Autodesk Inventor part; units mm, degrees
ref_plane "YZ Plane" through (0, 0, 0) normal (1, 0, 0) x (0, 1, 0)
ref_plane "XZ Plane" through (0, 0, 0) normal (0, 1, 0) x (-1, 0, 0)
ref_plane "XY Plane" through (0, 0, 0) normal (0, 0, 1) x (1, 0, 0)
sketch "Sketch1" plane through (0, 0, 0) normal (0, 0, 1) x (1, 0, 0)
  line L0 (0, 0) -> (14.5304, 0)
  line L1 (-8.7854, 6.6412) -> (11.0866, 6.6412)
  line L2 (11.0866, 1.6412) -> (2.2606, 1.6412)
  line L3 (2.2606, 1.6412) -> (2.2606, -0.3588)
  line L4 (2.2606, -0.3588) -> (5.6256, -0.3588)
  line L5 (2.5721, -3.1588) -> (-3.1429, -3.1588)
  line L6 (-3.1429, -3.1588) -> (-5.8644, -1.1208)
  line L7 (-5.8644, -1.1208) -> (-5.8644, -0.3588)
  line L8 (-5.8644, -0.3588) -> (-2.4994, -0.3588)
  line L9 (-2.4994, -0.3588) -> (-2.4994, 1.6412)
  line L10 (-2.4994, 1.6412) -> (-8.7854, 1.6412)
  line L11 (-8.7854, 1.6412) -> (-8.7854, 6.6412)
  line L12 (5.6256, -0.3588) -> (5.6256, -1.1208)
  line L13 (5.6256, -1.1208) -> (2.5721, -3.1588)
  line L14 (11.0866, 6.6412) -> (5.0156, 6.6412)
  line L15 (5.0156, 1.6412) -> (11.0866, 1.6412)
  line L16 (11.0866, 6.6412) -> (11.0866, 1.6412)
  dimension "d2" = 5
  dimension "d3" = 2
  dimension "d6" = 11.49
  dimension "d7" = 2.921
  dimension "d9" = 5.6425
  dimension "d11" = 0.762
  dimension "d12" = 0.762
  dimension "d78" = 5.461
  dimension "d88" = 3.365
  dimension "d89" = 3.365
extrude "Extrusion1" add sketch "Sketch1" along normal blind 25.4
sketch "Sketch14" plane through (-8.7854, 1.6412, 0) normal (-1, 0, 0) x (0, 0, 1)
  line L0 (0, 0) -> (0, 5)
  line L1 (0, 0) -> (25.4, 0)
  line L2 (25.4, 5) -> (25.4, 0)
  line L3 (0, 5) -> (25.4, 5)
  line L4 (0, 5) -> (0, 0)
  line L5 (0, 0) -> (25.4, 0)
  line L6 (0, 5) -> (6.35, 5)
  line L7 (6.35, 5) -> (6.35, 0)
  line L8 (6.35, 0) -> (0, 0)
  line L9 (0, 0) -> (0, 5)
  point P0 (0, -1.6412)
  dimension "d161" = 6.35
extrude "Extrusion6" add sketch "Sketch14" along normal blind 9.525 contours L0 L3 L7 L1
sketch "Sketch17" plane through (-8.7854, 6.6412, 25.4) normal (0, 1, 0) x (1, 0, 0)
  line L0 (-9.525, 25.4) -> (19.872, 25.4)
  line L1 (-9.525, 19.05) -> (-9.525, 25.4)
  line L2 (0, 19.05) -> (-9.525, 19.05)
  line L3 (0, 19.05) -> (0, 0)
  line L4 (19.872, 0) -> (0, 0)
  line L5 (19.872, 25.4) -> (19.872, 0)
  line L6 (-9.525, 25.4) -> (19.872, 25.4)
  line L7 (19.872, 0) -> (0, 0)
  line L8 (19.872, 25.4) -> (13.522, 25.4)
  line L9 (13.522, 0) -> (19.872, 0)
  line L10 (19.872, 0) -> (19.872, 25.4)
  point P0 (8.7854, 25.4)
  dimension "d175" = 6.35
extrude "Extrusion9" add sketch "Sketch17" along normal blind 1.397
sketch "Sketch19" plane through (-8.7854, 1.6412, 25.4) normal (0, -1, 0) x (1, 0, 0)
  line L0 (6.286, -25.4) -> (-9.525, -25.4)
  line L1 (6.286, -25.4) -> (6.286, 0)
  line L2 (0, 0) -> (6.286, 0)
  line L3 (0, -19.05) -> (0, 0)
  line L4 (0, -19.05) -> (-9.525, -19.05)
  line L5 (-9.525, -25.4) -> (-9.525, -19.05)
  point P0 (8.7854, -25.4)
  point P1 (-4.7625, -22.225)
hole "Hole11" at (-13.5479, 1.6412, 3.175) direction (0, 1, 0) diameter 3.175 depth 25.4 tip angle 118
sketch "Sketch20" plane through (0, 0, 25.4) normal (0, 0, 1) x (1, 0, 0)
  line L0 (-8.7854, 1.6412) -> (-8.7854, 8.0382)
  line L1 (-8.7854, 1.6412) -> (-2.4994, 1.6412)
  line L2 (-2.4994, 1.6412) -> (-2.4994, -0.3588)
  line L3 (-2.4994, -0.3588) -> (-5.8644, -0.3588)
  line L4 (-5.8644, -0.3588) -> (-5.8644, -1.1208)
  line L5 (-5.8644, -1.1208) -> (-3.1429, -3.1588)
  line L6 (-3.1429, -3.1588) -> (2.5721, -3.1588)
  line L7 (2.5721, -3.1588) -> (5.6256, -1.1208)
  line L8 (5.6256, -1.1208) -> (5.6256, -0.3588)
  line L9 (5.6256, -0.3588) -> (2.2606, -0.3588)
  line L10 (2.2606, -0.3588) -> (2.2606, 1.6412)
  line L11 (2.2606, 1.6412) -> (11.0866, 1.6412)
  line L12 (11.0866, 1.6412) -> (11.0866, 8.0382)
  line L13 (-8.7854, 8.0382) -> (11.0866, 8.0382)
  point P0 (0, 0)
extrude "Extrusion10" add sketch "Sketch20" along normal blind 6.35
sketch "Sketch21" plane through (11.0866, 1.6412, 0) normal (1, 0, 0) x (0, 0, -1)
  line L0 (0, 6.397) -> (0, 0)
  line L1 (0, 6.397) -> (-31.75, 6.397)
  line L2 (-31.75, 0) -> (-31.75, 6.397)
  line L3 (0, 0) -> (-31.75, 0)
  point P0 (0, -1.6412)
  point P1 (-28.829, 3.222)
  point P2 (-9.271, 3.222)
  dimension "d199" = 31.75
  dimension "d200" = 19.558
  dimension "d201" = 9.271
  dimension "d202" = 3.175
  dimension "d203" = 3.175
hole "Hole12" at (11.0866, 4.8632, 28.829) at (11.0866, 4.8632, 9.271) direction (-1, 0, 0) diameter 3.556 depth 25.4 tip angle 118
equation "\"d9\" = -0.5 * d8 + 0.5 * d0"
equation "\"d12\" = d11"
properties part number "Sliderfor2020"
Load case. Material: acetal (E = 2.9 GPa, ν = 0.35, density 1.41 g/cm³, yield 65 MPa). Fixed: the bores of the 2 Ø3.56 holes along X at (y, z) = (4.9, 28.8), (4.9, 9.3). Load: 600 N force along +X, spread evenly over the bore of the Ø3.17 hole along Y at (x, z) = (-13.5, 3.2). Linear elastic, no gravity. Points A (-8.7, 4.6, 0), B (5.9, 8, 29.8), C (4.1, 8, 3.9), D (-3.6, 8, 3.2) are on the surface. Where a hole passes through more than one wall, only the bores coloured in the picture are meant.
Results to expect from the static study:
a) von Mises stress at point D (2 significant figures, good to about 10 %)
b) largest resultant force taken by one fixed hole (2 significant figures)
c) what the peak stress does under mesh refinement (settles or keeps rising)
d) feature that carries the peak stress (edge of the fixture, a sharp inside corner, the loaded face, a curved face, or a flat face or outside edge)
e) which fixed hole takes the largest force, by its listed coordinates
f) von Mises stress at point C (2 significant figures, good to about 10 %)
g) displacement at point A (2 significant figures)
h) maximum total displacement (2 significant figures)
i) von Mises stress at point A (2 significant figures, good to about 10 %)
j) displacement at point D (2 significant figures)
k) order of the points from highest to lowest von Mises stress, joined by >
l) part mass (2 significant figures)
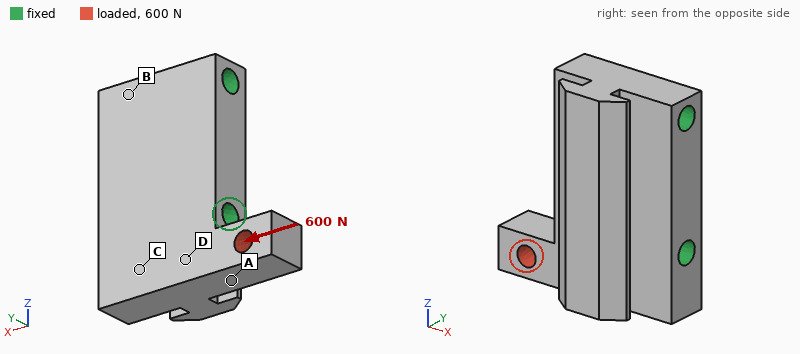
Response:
11 MPa
610 N
keeps rising
edge of the fixture
(4.9, 9.3)
5.7 MPa
0.075 mm
0.13 mm
19 MPa
0.030 mm
A > D > C > B
7.2 g
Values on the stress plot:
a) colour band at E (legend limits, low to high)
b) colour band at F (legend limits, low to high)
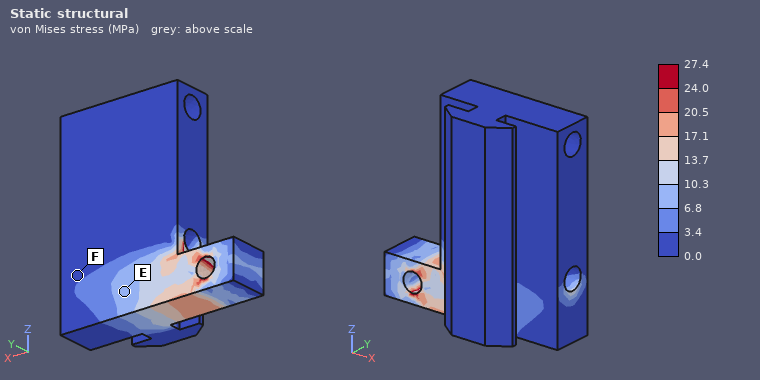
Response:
6.8 to 10.3 MPa
0.0 to 3.4 MPa
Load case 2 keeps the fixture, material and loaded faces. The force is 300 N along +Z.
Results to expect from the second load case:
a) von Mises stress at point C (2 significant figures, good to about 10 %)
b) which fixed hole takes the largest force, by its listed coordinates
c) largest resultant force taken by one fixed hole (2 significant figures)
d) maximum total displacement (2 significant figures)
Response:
4.2 MPa
(4.9, 9.3)
300 N
0.36 mm
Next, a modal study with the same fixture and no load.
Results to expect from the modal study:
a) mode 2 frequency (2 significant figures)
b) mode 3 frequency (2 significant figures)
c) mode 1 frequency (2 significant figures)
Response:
7600 Hz
12 kHz
6300 Hz
